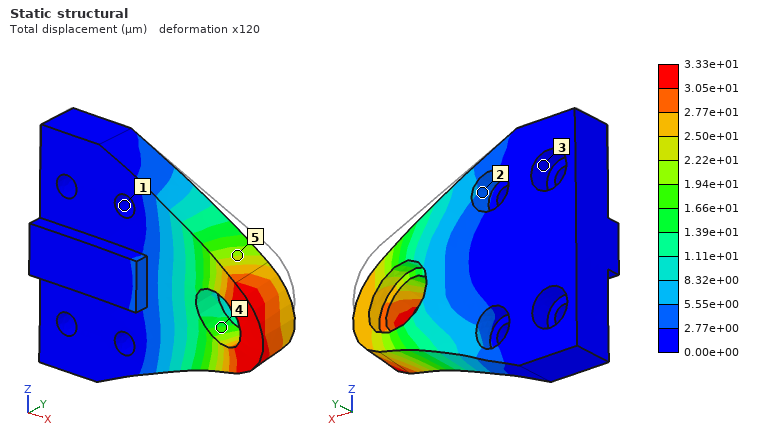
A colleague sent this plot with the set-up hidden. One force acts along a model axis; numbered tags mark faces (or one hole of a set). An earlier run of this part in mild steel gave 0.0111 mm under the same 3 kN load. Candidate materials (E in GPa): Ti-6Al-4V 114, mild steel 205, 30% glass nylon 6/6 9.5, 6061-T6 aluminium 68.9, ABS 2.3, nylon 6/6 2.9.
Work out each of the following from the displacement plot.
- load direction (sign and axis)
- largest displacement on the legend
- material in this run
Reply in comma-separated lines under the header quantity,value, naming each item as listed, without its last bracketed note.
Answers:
quantity,value
load direction,-Z
largest displacement on the legend,3.33e+01 µm
material in this run,6061-T6 aluminium
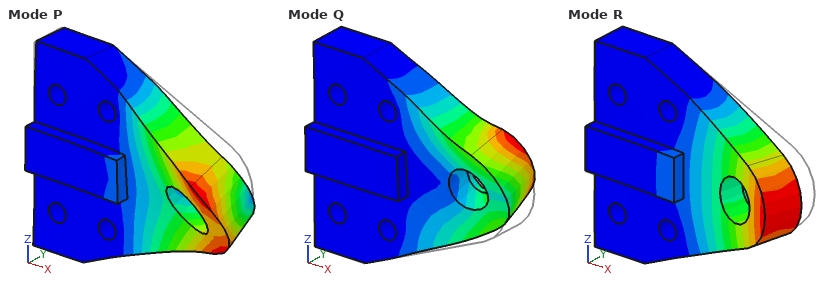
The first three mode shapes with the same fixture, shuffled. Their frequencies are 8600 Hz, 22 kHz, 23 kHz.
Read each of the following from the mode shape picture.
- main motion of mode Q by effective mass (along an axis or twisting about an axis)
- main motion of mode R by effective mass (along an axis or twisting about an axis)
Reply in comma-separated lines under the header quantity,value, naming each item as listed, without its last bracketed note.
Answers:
quantity,value
main motion of mode Q by effective mass,along Z
main motion of mode R by effective mass,along Y
